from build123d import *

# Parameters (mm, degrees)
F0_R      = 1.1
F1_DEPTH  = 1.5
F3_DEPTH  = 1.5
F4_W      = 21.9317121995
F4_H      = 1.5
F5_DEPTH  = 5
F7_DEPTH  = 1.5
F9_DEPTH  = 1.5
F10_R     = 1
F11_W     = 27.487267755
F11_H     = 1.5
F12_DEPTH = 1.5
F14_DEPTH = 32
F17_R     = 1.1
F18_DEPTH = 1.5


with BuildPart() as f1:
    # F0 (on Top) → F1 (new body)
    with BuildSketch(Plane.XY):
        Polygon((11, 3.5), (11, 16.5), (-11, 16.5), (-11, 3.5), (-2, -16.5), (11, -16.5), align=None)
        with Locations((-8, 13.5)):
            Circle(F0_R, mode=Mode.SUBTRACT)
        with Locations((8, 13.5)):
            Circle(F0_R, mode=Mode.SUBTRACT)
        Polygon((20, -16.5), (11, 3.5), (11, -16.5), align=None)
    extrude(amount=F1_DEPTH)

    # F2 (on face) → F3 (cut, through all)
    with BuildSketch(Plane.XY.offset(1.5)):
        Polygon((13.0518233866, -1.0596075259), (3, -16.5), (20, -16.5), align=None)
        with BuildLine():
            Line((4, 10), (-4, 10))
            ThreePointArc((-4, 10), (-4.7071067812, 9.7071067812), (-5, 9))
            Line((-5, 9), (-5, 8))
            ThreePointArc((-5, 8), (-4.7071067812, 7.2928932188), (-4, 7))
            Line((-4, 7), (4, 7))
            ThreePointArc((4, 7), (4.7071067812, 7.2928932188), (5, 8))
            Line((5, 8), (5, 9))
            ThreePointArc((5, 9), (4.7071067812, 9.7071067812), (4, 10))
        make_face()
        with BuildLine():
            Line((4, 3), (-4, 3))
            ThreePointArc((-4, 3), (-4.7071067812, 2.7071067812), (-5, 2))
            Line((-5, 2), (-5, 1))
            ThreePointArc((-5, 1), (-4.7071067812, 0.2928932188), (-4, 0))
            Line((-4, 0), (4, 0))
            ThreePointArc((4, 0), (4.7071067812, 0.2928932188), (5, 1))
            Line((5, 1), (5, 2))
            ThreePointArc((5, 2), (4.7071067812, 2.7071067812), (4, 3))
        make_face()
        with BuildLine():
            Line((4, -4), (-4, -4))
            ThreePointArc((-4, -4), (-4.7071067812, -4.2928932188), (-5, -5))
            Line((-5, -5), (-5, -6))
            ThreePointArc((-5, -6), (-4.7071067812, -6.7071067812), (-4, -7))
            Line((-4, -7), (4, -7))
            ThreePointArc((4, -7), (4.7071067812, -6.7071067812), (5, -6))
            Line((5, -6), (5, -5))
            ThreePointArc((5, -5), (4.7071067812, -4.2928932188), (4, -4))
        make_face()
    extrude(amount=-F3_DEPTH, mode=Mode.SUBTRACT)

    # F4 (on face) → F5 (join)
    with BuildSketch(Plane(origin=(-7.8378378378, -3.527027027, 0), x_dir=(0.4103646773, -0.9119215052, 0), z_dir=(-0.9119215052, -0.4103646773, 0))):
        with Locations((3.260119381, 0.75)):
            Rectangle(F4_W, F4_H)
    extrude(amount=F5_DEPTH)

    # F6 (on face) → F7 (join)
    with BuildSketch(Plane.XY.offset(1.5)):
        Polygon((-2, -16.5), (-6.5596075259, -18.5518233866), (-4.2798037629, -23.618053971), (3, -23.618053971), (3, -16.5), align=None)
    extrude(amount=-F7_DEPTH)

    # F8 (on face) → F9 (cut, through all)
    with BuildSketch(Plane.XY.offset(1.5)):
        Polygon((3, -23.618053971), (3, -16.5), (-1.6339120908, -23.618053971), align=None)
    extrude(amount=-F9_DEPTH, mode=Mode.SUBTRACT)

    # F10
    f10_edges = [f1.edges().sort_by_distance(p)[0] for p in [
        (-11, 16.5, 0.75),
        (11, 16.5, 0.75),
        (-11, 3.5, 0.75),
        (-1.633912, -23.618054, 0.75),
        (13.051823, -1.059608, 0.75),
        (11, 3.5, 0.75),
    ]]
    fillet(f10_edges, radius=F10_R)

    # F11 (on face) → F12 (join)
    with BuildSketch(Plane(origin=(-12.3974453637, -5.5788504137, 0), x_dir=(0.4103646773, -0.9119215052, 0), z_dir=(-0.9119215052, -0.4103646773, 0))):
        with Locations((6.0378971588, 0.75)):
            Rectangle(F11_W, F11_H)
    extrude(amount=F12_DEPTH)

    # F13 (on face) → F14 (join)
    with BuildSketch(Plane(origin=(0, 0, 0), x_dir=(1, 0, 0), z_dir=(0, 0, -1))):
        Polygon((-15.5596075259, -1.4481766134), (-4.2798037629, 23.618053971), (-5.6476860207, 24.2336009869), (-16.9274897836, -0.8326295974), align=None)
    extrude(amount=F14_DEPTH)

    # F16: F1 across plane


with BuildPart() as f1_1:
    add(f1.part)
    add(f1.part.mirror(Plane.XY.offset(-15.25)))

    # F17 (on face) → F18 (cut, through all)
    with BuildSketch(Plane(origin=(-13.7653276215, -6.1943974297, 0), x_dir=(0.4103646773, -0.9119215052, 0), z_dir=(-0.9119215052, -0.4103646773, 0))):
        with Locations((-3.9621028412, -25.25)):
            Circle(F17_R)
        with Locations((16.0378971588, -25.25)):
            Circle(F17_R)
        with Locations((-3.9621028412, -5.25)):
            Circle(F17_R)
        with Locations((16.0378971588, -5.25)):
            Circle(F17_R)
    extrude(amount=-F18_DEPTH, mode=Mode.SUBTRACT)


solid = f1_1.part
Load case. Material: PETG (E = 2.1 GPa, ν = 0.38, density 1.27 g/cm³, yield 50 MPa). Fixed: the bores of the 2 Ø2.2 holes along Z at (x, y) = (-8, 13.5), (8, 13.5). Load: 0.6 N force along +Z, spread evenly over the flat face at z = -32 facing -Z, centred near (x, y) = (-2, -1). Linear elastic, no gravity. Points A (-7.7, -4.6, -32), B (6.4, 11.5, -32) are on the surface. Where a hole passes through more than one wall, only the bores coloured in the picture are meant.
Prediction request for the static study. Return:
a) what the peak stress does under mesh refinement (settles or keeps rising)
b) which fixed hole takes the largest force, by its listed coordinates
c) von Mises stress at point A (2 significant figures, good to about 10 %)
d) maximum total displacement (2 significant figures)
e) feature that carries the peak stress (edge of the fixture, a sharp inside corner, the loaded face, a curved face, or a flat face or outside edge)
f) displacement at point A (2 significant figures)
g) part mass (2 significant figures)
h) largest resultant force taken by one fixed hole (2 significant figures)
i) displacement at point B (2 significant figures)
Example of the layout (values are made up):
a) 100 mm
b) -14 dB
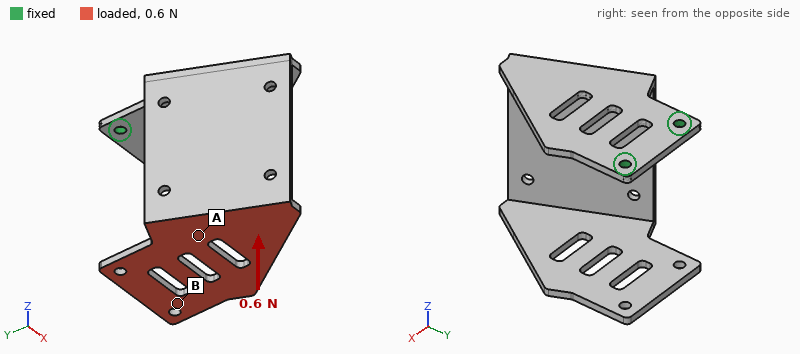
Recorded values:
a) keeps rising
b) (-8, 13.5)
c) 0.58 MPa
d) 0.71 mm
e) edge of the fixture
f) 0.38 mm
g) 4.2 g
h) 0.36 N
i) 0.61 mm
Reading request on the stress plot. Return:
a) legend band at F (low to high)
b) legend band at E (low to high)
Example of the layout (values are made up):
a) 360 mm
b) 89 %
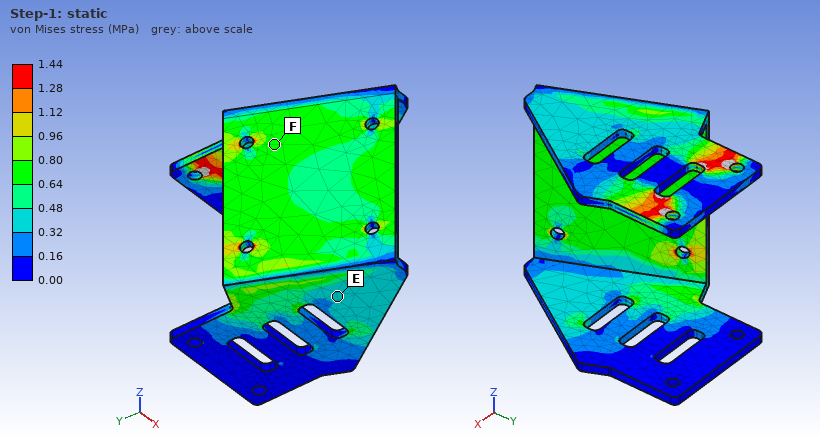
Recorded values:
a) 0.64 to 0.80 MPa
b) 0.32 to 0.48 MPa
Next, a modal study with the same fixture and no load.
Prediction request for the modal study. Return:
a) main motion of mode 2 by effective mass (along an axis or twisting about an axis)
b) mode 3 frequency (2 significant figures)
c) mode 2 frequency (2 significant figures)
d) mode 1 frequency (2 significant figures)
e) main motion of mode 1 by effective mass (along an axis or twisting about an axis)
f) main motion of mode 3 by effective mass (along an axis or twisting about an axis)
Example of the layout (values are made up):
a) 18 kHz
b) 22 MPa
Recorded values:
a) along X
b) 200 Hz
c) 87 Hz
d) 60 Hz
e) along Y
f) along Z
